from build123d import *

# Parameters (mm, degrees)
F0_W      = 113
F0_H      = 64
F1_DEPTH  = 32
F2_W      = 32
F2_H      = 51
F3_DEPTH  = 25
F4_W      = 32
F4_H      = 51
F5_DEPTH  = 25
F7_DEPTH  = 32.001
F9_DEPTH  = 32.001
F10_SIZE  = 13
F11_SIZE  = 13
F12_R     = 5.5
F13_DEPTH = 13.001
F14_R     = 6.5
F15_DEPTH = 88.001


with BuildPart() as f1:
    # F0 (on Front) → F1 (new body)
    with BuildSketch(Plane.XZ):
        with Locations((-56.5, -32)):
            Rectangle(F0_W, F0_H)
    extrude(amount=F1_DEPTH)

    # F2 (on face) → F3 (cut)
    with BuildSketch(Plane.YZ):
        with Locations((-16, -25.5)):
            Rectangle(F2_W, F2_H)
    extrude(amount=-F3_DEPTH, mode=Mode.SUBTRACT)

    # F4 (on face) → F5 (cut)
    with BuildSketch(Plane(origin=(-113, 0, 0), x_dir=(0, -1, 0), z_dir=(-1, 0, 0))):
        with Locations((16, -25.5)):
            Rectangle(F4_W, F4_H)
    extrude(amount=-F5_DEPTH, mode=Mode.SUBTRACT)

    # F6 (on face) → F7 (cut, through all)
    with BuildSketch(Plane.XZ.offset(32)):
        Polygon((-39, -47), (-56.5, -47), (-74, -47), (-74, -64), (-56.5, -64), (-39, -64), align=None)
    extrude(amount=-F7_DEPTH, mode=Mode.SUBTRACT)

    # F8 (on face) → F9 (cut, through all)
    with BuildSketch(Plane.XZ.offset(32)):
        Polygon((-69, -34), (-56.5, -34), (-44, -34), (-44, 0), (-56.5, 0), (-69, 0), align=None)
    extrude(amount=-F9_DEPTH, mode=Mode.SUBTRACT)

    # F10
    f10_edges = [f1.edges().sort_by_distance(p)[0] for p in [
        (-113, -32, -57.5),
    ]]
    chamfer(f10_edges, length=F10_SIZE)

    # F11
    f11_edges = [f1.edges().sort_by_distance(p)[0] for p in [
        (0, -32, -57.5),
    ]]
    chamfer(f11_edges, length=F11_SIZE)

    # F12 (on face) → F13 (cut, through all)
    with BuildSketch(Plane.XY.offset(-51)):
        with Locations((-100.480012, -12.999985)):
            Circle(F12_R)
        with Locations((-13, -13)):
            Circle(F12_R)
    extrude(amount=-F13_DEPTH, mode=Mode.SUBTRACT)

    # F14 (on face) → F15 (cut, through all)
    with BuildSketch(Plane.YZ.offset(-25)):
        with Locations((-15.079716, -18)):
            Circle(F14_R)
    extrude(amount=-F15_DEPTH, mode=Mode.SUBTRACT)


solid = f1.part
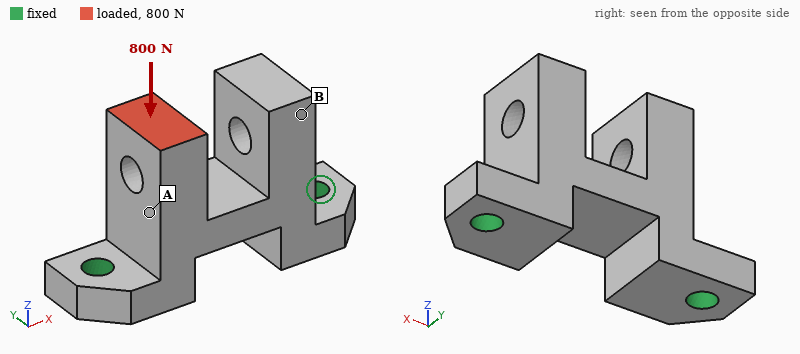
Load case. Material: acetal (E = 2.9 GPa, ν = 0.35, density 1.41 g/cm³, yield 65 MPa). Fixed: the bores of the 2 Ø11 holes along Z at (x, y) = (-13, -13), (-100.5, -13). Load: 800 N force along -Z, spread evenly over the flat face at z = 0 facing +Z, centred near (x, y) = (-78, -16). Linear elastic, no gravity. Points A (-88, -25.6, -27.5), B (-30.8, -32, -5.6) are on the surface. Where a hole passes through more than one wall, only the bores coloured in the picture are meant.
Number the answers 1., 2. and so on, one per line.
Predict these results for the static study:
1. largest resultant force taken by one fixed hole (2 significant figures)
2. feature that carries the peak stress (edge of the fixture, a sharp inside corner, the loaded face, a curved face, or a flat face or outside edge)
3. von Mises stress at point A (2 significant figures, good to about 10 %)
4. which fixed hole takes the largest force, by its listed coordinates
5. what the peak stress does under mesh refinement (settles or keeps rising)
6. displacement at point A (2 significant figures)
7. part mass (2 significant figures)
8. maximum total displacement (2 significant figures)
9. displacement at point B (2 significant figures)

1. 720 N
2. edge of the fixture
3. 2.0 MPa
4. (-100.5, -13)
5. keeps rising
6. 75 µm
7. 130 g
8. 96 µm
9. 32 µm
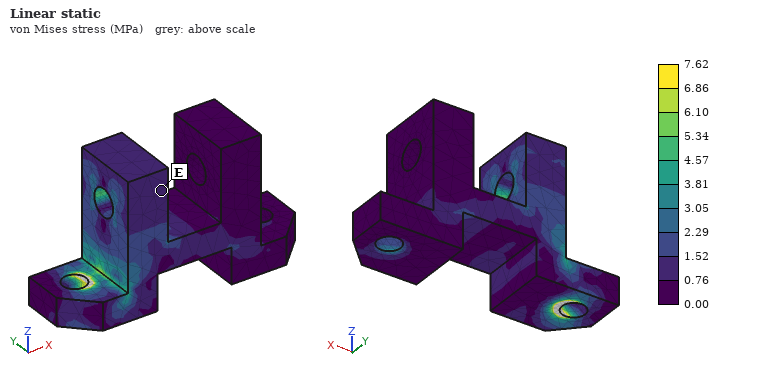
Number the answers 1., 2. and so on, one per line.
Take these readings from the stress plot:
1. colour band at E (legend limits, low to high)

1. 0.76 to 1.52 MPa
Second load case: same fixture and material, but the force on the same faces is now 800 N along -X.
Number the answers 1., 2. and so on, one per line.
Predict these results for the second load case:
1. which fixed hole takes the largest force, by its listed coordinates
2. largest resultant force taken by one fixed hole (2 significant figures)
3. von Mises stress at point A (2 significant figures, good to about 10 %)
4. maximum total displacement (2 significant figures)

1. (-13, -13)
2. 1.2 kN
3. 15 MPa
4. 0.82 mm
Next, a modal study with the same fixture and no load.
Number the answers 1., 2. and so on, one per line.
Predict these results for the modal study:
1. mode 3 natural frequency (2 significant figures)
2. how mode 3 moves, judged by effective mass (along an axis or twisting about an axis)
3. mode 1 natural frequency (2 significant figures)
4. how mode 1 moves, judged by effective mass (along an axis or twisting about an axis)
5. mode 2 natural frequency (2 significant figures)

1. 1500 Hz
2. along X
3. 760 Hz
4. along Y
5. 1300 Hz
